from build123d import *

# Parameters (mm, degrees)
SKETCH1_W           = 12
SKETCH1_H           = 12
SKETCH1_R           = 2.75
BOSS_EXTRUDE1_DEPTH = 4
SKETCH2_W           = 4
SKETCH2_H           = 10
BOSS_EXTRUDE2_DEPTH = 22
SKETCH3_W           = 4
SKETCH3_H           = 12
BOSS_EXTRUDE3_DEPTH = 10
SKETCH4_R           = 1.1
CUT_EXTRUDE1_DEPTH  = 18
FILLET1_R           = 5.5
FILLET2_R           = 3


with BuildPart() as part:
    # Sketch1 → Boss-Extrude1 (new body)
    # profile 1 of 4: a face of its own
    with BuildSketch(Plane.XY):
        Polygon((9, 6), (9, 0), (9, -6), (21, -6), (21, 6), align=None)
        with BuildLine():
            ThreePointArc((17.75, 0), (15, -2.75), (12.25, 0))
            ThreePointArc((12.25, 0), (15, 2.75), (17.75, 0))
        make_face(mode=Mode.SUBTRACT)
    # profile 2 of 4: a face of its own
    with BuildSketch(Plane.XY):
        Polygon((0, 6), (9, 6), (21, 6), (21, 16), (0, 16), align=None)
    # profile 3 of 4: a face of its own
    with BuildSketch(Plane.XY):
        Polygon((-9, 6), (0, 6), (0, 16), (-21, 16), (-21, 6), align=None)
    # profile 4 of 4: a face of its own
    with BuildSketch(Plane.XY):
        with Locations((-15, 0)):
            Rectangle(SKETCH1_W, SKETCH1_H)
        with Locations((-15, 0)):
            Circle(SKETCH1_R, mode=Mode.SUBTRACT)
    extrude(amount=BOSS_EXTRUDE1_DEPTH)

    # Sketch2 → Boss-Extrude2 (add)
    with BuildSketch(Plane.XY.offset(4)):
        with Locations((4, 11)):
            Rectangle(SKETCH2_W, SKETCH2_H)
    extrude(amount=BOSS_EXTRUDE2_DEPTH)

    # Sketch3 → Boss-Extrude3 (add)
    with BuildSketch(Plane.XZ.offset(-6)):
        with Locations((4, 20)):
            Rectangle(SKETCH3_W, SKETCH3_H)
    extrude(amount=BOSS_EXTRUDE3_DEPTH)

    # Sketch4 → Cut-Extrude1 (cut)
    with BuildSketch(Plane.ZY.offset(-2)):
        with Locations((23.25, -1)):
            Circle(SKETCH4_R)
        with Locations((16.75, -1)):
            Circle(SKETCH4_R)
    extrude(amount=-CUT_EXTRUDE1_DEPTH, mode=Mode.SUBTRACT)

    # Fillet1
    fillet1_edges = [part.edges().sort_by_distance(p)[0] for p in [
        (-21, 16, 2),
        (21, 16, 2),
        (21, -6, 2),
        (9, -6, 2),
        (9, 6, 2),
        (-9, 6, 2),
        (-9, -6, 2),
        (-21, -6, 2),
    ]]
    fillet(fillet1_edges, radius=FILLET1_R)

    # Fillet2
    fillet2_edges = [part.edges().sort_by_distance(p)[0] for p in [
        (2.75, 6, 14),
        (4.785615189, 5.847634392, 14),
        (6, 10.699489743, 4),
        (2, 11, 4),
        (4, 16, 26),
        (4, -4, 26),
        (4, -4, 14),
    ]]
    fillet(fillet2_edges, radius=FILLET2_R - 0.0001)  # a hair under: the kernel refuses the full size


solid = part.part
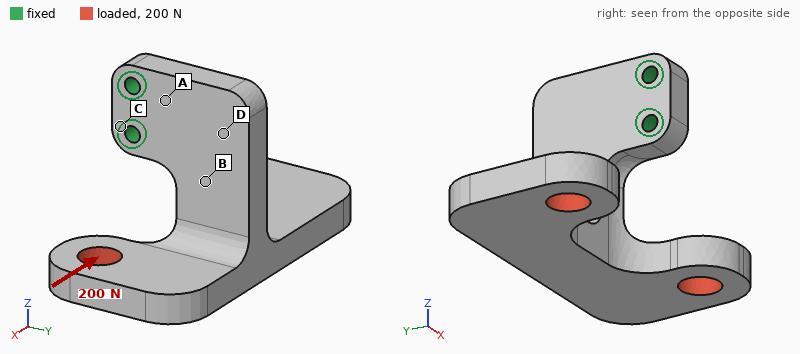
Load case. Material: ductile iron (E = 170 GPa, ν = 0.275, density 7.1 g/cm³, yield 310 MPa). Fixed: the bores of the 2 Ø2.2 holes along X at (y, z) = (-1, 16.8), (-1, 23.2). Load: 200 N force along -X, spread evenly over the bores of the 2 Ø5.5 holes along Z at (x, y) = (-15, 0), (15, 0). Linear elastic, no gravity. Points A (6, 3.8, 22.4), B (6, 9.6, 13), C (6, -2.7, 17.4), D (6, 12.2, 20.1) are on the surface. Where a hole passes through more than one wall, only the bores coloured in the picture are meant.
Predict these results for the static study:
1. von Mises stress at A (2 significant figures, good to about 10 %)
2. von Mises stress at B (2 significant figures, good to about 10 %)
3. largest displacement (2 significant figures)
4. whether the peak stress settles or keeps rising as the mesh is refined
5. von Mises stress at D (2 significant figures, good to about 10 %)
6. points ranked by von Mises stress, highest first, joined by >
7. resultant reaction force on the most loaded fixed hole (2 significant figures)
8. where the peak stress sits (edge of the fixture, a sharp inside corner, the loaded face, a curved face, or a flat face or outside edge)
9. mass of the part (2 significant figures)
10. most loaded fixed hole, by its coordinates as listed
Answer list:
60 MPa
110 MPa
0.15 mm
keeps rising
37 MPa
B > A > D > C
460 N
edge of the fixture
28 g
(-1, 16.8)
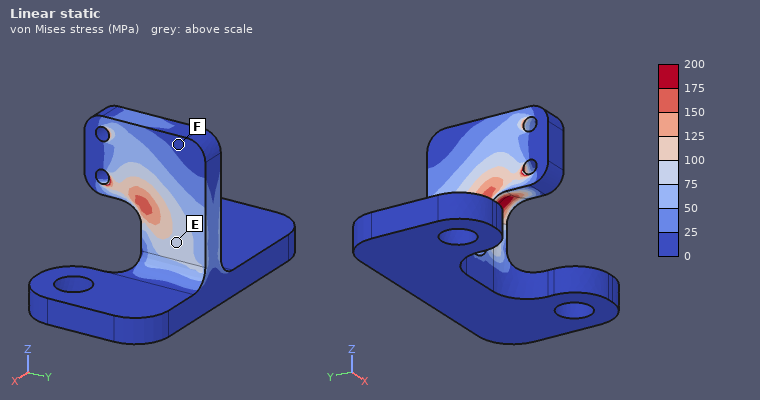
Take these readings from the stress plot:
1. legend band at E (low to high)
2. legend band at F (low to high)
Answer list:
75 to 100 MPa
0 to 25 MPa
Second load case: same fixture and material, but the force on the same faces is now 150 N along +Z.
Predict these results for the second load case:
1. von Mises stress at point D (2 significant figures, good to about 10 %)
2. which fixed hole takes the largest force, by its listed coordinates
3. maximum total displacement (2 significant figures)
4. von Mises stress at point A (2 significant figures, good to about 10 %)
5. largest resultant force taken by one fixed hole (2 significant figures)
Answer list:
14 MPa
(-1, 16.8)
70 µm
7.0 MPa
100 N
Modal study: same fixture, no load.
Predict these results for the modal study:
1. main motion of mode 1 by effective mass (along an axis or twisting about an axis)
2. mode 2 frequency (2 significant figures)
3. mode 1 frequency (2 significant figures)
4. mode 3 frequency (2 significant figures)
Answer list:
along X
1800 Hz
1500 Hz
4100 Hz
